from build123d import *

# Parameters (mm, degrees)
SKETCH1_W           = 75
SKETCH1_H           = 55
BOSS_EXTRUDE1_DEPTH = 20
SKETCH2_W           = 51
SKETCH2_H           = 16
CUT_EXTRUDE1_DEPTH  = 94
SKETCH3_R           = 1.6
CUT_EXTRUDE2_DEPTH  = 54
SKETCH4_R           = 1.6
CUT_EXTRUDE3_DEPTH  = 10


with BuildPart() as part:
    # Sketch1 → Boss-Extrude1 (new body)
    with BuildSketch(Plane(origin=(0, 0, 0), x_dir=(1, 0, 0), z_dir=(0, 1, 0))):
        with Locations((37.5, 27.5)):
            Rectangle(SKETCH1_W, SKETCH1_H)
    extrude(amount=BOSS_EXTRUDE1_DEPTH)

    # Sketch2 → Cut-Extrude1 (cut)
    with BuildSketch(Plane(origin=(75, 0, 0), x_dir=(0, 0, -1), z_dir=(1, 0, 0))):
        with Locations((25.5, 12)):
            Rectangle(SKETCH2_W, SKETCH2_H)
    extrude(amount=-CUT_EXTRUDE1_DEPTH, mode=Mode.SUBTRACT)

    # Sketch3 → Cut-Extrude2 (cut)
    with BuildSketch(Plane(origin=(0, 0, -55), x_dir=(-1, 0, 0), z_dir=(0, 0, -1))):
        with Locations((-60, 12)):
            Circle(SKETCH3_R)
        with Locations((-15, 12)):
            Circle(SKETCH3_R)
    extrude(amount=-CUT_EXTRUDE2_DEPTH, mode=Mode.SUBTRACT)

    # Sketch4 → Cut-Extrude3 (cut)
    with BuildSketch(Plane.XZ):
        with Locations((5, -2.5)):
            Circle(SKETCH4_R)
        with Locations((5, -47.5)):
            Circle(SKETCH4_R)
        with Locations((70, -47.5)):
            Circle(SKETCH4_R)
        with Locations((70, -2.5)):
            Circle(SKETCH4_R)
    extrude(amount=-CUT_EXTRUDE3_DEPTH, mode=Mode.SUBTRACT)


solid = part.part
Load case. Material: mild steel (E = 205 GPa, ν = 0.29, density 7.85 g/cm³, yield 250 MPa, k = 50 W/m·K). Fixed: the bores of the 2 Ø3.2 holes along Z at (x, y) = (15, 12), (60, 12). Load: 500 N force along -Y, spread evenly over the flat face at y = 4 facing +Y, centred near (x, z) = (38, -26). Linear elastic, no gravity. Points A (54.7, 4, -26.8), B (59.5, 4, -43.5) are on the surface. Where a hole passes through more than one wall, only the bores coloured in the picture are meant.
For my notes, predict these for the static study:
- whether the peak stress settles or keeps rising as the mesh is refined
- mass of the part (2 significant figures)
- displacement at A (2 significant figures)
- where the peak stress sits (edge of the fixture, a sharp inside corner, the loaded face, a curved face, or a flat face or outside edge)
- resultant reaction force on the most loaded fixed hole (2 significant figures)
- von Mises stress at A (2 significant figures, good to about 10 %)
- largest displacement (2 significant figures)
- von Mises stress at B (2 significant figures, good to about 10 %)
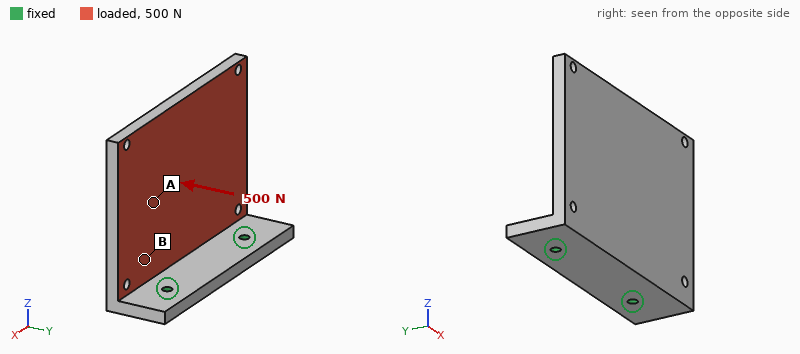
keeps rising
170 g
0.098 mm
edge of the fixture
260 N
16 MPa
0.23 mm
41 MPa
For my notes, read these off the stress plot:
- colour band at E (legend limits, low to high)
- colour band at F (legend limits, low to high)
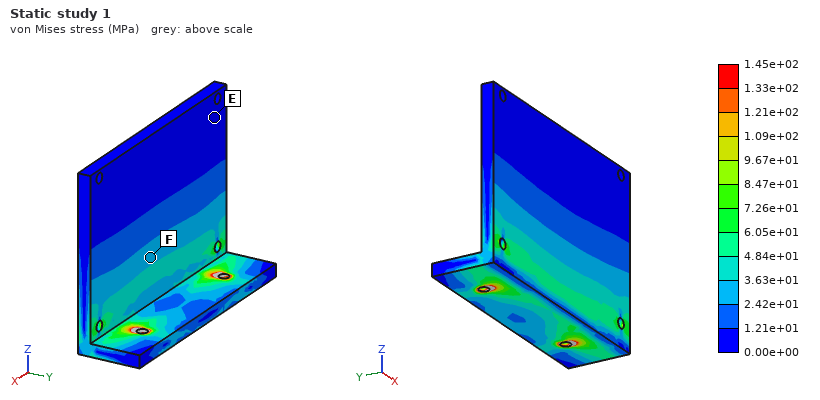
0.00e+00 to 1.21e+01 MPa
2.42e+01 to 3.63e+01 MPa
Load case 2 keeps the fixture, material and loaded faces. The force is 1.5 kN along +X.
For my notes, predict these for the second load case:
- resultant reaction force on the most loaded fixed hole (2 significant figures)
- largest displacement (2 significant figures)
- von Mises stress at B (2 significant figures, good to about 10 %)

1.2 kN
60 µm
33 MPa
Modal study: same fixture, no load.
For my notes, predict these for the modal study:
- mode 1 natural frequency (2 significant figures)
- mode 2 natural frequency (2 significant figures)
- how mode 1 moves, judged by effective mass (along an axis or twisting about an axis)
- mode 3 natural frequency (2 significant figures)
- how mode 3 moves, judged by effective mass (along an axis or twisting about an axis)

840 Hz
1900 Hz
along Y
3600 Hz
along X
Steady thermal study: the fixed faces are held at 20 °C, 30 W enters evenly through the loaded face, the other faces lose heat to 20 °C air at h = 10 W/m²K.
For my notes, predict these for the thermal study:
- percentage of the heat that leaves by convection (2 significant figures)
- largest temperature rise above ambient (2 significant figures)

12 %
79 K
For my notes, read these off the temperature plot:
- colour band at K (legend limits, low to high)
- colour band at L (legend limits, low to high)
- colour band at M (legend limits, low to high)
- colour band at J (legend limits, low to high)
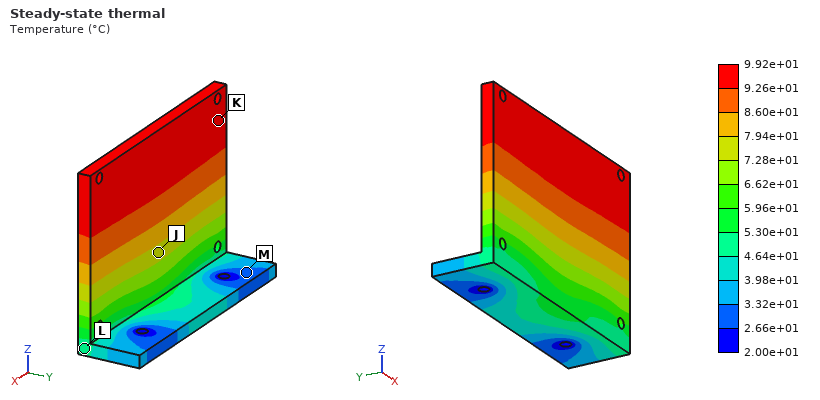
9.26e+01 to 9.92e+01 °C
4.64e+01 to 5.30e+01 °C
2.66e+01 to 3.32e+01 °C
7.28e+01 to 7.94e+01 °C
